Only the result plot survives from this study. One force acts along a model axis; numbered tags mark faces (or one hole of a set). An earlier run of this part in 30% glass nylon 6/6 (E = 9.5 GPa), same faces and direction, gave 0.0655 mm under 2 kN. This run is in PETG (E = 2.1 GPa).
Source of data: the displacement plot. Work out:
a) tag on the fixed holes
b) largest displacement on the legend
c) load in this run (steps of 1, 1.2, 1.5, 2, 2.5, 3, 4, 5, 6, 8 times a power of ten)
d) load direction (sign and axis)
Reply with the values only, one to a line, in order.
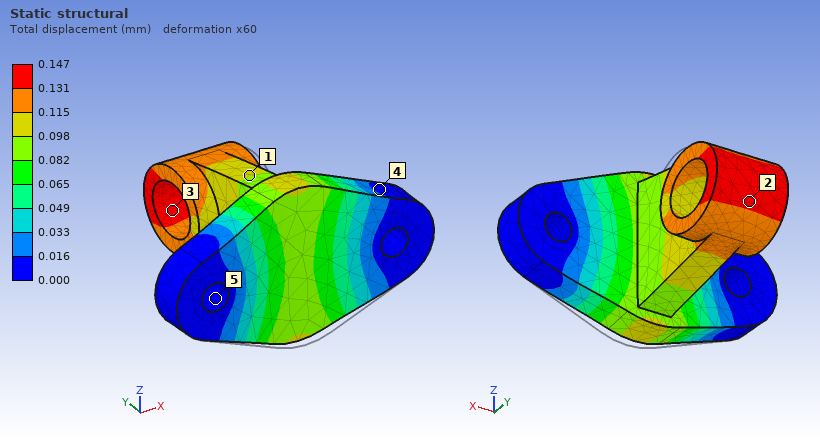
5
0.147 mm
1 kN
+Y
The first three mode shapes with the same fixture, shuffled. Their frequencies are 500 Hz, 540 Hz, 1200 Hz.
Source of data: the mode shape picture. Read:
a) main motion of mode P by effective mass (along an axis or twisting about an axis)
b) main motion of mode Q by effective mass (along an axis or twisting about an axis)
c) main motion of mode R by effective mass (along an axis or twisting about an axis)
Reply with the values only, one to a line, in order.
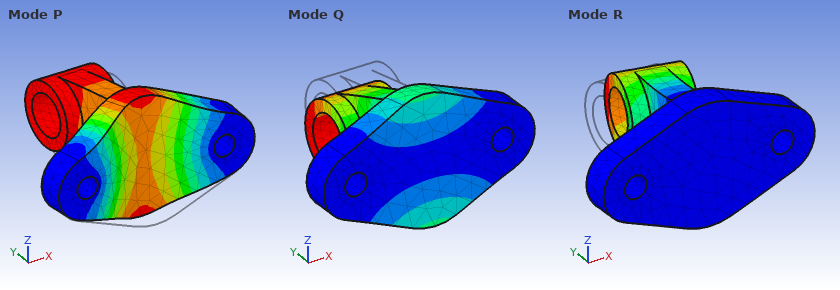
along Y
along Z
along X
